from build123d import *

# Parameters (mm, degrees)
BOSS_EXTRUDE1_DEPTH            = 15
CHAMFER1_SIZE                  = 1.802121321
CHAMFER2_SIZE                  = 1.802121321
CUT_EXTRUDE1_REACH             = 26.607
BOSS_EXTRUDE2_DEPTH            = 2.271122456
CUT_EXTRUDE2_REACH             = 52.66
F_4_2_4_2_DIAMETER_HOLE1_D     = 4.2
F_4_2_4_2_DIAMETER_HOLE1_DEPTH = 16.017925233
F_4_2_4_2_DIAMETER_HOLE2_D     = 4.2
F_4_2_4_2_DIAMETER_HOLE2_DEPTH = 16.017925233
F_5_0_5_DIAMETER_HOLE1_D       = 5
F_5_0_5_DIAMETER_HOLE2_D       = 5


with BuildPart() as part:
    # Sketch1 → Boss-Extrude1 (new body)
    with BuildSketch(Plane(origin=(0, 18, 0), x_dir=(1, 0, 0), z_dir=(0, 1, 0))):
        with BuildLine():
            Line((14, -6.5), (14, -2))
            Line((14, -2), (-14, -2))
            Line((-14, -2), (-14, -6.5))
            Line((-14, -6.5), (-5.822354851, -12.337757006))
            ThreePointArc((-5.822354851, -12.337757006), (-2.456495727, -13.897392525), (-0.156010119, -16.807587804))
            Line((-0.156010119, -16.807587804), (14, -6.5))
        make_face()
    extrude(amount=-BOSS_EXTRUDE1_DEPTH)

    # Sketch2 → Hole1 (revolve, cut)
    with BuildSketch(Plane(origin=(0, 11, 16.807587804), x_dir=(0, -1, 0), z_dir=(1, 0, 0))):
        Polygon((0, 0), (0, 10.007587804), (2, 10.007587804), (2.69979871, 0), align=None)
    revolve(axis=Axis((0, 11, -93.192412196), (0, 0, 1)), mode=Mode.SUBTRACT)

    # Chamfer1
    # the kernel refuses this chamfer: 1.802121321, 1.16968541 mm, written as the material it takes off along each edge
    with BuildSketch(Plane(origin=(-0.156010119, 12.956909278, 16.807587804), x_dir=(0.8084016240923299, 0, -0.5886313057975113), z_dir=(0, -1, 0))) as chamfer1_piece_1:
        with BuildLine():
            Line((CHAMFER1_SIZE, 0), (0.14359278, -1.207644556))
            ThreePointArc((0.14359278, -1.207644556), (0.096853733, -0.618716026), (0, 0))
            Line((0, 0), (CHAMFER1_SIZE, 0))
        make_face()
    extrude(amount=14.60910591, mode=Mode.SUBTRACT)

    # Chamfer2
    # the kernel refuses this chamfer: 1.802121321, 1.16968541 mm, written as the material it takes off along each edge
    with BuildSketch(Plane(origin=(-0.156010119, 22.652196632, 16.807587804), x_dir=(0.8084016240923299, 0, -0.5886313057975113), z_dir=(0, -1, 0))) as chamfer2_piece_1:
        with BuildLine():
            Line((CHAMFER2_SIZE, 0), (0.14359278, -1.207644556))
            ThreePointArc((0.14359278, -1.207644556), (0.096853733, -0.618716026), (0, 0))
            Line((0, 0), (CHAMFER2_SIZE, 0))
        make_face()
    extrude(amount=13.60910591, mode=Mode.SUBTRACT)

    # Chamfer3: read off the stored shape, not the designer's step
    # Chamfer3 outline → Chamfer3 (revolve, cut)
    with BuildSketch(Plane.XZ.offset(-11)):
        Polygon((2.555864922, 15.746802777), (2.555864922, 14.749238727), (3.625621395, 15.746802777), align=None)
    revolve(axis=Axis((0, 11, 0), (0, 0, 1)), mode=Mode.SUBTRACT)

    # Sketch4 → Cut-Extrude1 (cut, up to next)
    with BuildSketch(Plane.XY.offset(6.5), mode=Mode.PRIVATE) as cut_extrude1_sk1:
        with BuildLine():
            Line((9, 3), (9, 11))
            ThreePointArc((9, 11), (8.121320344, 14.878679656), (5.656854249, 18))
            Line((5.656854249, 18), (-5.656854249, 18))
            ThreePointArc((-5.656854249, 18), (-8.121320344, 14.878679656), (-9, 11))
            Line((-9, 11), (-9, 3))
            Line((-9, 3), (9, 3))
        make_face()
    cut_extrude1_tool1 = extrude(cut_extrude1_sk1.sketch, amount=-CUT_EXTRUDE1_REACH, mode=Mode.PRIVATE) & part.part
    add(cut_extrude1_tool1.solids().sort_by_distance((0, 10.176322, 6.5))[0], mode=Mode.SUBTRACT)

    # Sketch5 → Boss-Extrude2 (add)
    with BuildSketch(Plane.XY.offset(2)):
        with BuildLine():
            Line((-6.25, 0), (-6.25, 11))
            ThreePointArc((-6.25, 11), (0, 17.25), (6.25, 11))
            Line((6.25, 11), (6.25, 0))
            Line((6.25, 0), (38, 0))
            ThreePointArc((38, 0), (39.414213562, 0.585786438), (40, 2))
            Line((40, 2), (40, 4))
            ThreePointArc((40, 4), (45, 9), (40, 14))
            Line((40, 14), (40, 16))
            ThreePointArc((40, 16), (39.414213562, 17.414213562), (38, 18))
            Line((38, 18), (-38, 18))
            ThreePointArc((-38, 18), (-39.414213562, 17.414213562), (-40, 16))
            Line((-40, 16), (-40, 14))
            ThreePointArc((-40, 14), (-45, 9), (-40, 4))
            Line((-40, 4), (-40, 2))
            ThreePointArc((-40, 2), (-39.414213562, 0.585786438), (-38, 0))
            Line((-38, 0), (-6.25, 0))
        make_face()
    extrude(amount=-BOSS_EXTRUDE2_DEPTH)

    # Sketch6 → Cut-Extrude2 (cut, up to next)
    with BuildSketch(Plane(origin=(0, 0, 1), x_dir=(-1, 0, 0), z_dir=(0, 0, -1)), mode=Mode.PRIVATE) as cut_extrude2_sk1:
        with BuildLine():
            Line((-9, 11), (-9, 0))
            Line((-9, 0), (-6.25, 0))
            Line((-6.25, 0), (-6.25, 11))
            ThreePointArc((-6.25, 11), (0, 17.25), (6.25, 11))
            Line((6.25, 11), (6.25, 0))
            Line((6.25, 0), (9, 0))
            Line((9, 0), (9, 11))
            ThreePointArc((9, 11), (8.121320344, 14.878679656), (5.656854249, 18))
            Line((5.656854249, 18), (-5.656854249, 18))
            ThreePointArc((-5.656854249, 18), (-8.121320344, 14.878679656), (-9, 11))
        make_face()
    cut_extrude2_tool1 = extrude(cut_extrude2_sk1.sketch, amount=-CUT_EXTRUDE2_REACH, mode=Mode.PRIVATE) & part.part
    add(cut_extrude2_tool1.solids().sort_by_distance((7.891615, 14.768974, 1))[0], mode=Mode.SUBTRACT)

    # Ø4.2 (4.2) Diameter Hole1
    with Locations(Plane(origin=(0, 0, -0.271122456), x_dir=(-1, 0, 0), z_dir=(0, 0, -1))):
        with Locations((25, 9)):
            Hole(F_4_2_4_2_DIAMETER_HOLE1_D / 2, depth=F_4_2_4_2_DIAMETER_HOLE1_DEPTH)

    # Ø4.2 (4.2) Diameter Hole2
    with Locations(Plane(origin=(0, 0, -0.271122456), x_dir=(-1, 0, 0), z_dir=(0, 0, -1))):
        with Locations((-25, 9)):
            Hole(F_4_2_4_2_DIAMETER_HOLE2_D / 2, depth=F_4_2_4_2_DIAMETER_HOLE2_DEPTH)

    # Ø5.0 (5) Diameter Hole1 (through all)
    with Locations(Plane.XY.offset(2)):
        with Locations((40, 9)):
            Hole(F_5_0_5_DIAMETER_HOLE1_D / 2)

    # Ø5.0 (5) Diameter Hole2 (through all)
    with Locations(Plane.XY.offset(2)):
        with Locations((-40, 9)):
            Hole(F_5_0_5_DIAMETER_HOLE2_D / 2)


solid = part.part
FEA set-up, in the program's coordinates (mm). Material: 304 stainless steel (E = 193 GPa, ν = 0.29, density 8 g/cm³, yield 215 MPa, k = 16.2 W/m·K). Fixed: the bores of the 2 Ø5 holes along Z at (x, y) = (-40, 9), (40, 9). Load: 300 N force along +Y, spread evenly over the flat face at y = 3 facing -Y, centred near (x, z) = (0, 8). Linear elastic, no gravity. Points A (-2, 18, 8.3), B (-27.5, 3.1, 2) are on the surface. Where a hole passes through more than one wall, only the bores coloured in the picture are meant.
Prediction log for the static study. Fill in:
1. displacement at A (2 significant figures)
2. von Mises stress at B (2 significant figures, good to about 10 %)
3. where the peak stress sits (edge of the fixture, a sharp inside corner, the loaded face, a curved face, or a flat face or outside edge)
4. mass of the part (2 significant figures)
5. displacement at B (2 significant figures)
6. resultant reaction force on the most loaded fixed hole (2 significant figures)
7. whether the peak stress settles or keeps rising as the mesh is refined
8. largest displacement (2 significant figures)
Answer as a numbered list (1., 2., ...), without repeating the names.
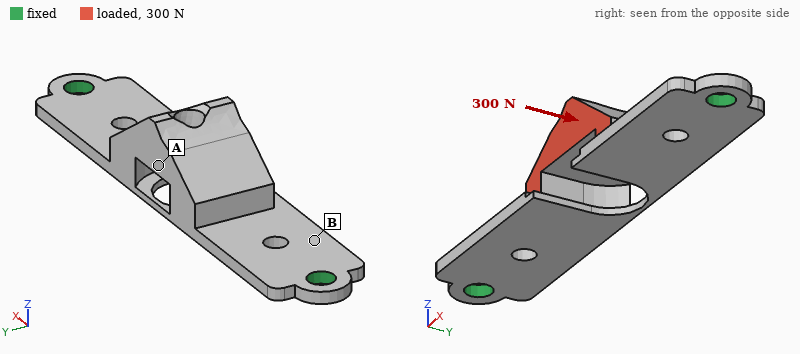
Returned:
1. 0.074 mm
2. 70 MPa
3. edge of the fixture
4. 43 g
5. 0.017 mm
6. 170 N
7. keeps rising
8. 0.11 mm
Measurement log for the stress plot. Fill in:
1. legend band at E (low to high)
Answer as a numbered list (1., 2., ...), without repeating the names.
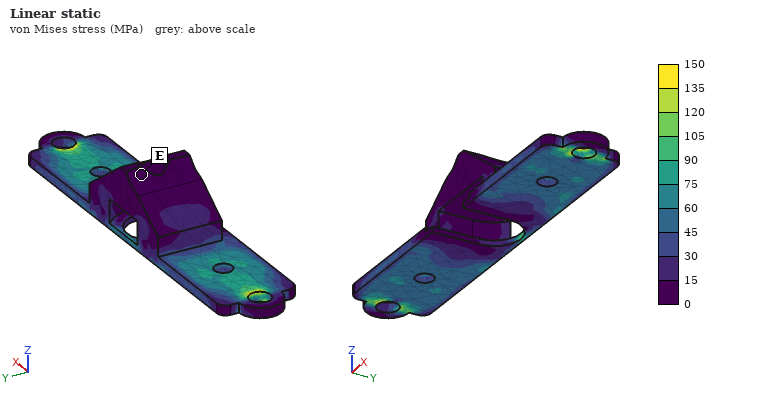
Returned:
1. 0 to 15 MPa
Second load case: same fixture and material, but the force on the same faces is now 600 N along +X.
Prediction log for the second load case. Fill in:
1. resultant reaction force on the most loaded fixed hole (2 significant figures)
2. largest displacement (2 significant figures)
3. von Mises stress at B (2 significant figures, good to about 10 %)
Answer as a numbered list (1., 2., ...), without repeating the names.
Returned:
1. 320 N
2. 23 µm
3. 15 MPa
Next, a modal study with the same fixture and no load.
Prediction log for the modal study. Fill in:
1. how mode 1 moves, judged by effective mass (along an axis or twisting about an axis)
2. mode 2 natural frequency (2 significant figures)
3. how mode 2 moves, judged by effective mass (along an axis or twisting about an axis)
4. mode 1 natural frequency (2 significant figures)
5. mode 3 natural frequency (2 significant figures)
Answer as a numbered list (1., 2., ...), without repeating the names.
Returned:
1. along Z
2. 2200 Hz
3. along Y
4. 1800 Hz
5. 4000 Hz
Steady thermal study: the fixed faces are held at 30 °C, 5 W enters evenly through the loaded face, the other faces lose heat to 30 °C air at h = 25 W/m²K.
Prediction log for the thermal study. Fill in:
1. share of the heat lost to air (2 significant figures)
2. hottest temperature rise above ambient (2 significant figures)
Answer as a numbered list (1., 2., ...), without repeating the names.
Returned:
1. 68 %
2. 67 K
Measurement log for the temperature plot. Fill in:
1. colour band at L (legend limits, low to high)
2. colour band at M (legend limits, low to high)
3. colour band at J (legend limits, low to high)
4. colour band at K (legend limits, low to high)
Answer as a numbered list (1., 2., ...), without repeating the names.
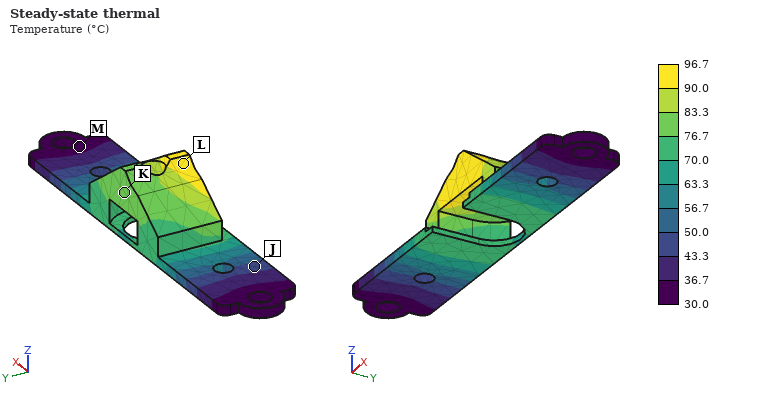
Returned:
1. 90.0 to 96.7 °C
2. 30.0 to 36.7 °C
3. 43.3 to 50.0 °C
4. 76.7 to 83.3 °C
